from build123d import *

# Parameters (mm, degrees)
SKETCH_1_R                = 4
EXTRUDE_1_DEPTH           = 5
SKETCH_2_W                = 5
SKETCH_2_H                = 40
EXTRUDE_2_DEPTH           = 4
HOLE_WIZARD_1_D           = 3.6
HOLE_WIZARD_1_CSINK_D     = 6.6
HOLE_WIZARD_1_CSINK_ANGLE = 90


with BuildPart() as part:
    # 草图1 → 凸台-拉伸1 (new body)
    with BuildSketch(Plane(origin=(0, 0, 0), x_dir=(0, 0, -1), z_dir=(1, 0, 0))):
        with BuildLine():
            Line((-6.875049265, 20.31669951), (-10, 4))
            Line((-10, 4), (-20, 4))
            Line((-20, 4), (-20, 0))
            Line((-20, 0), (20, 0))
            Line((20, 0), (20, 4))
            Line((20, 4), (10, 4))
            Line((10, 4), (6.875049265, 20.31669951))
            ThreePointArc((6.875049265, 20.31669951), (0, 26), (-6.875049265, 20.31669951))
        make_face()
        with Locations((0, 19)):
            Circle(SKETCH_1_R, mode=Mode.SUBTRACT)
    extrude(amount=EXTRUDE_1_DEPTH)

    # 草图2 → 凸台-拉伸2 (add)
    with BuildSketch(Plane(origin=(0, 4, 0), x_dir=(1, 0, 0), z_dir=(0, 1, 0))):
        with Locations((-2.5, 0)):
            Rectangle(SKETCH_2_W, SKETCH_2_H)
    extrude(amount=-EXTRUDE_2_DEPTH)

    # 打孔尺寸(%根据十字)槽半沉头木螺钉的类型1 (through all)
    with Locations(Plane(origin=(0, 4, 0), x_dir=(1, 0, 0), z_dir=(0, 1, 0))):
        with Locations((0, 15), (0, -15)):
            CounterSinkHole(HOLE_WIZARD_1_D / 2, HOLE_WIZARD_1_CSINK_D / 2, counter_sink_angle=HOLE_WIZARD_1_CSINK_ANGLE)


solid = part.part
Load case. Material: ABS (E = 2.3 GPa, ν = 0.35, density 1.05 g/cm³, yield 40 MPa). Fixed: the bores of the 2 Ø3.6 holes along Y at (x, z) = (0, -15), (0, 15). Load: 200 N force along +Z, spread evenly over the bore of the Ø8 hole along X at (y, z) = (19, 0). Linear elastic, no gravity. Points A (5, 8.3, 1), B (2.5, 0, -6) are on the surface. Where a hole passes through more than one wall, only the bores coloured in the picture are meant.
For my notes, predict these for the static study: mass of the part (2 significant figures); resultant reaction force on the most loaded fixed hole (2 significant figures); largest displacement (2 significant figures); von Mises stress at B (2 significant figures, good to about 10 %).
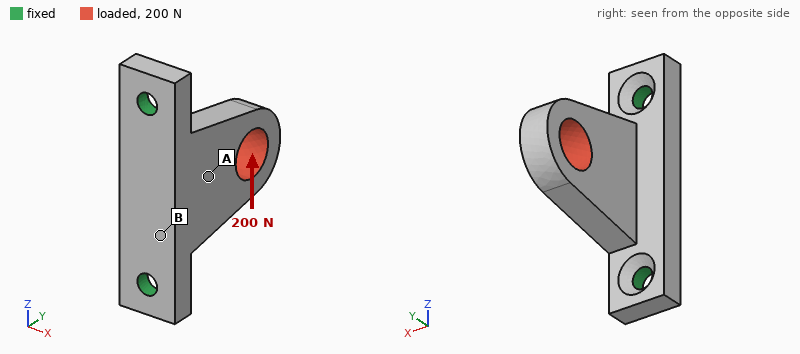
3.0 g
170 N
0.36 mm
7.8 MPa
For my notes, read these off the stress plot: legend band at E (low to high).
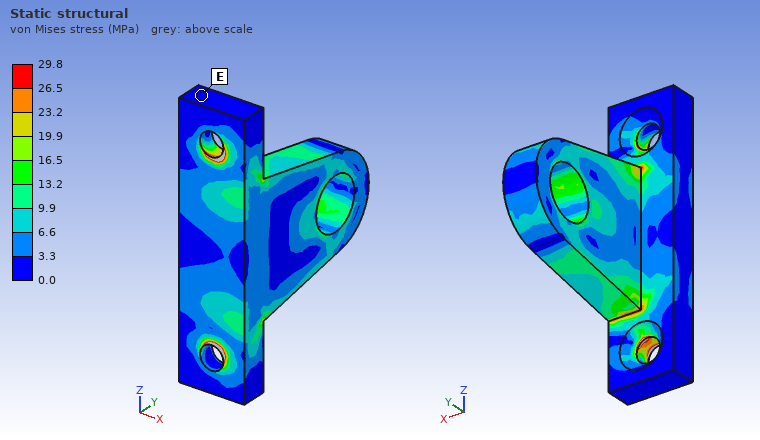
0.0 to 3.3 MPa
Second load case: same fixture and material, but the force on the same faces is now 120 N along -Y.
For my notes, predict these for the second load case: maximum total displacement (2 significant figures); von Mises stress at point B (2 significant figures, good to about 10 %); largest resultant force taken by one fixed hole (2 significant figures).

0.19 mm
2.8 MPa
73 N
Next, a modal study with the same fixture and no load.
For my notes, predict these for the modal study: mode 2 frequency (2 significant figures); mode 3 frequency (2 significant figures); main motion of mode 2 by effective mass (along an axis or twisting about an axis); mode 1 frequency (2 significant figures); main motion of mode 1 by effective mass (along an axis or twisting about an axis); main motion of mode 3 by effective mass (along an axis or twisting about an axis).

5100 Hz
5400 Hz
along Z
1600 Hz
along X
along Y
